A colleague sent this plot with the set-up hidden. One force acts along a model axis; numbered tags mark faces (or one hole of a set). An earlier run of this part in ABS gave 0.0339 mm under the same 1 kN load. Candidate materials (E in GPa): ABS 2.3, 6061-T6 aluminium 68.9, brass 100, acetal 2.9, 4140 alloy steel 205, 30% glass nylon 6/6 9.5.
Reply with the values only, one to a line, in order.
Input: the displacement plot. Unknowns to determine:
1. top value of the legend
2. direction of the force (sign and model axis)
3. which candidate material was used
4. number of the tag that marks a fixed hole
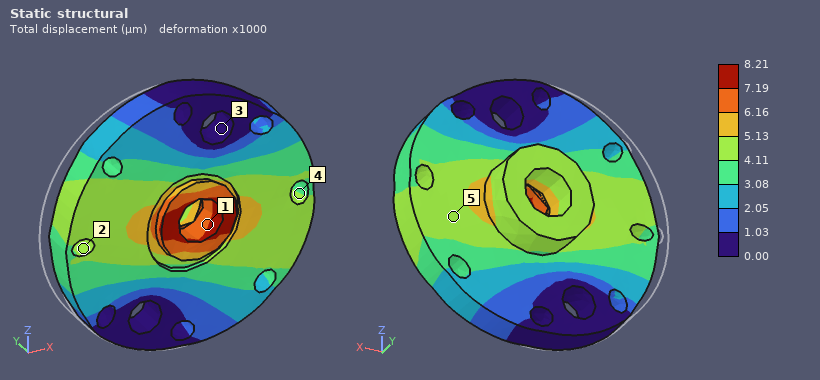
8.21 µm
+X
30% glass nylon 6/6
3
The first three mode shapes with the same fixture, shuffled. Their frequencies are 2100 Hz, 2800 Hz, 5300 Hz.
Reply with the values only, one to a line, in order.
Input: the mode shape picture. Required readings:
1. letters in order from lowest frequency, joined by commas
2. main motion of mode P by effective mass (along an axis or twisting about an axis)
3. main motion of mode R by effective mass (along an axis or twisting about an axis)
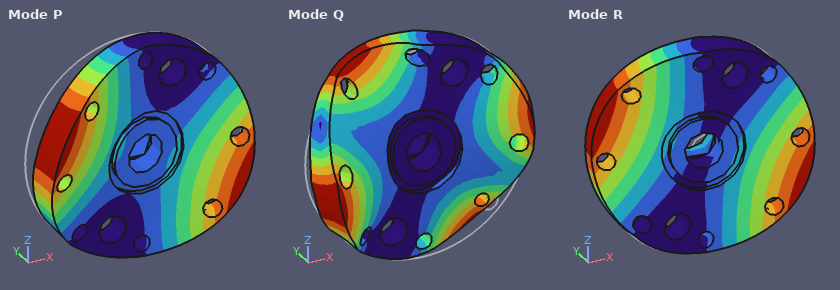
R, P, Q
along Y
twisting about Z
